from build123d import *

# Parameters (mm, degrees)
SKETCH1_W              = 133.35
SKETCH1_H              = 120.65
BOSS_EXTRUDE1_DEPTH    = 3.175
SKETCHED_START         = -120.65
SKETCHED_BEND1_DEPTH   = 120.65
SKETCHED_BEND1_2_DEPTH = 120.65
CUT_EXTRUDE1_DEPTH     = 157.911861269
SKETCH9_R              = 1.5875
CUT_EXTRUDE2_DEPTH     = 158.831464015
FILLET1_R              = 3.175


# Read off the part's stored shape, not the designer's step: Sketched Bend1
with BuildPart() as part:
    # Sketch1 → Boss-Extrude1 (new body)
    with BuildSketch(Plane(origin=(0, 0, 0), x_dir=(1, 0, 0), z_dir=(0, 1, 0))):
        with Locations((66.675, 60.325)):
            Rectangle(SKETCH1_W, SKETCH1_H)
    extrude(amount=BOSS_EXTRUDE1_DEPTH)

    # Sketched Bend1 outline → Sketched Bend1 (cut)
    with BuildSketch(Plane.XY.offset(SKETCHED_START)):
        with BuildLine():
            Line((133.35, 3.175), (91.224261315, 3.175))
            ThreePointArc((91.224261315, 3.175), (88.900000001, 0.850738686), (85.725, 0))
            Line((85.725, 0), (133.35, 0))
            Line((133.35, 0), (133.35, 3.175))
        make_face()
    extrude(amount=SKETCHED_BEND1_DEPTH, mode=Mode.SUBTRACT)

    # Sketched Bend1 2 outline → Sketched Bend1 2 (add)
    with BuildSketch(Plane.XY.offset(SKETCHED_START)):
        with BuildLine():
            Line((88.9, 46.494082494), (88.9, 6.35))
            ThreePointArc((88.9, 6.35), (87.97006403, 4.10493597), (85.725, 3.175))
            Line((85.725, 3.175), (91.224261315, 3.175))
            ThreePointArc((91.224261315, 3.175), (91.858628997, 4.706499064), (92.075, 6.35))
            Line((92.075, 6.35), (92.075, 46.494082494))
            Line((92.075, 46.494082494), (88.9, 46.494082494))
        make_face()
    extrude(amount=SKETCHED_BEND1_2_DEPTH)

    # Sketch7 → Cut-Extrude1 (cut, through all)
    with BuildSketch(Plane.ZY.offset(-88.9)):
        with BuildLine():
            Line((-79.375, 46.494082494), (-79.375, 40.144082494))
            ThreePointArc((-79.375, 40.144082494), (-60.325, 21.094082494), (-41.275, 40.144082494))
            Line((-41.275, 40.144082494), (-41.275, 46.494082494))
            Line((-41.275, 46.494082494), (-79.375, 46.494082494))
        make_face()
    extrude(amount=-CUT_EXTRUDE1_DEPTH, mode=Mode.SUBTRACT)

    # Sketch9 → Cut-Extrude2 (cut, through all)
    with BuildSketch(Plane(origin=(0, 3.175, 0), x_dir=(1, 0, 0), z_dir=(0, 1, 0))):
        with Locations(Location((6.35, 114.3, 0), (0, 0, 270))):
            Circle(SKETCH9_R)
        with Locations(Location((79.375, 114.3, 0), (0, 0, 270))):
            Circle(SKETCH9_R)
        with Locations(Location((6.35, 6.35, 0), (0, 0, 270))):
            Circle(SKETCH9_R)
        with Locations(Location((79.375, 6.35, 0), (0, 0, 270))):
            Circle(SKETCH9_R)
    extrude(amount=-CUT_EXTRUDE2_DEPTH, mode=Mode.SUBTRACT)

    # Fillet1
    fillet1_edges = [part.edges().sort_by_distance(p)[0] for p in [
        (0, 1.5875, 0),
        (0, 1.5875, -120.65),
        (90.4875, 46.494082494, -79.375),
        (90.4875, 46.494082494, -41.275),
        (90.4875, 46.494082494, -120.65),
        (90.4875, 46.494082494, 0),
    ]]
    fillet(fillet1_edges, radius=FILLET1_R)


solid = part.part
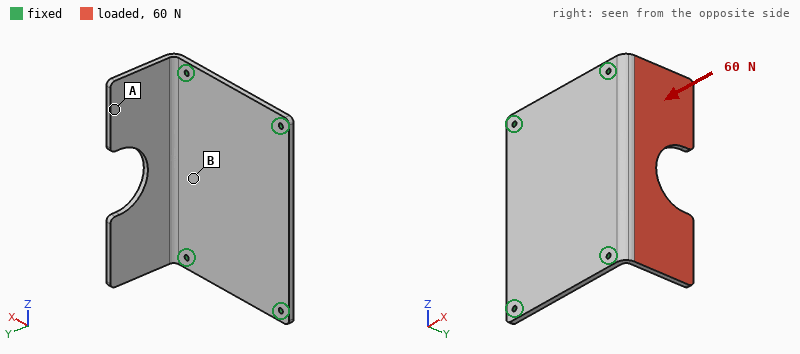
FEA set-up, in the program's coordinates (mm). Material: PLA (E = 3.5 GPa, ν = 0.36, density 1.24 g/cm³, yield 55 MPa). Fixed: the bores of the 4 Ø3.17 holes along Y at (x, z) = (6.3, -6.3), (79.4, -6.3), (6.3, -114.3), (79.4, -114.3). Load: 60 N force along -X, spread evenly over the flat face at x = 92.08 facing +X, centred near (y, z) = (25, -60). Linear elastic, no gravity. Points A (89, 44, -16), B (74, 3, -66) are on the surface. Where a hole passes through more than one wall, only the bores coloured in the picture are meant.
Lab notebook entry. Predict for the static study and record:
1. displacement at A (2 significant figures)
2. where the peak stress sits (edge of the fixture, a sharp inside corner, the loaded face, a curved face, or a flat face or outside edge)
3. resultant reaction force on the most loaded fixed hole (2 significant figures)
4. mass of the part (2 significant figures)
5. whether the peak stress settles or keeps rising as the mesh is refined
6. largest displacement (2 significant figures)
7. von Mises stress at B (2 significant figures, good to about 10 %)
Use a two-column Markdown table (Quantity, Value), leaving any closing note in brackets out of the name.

| Quantity | Value |
|---|---|
| displacement at A | 1.3 mm |
| where the peak stress sits | edge of the fixture |
| resultant reaction force on the most loaded fixed hole | 21 N |
| mass of the part | 60 g |
| whether the peak stress settles or keeps rising as the mesh is refined | keeps rising |
| largest displacement | 1.5 mm |
| von Mises stress at B | 3.4 MPa |
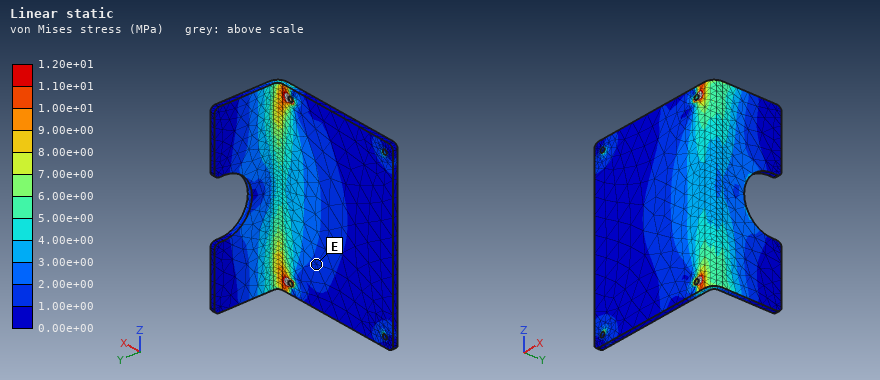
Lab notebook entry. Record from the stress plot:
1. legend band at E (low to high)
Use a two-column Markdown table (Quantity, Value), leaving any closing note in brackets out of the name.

| Quantity | Value |
|---|---|
| legend band at E | 1.00e+00 to 2.00e+00 MPa |
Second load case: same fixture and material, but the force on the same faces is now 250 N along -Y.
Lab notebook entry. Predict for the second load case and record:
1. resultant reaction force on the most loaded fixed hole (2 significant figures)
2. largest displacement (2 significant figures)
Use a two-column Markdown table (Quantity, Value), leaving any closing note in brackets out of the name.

| Quantity | Value |
|---|---|
| resultant reaction force on the most loaded fixed hole | 160 N |
| largest displacement | 1.8 mm |
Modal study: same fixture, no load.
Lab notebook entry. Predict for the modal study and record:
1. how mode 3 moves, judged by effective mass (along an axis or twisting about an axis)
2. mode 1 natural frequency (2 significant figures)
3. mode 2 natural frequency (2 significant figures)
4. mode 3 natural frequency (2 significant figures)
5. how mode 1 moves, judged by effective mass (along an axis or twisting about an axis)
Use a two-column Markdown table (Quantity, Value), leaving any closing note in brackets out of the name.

| Quantity | Value |
|---|---|
| how mode 3 moves, judged by effective mass | along Y |
| mode 1 natural frequency | 310 Hz |
| mode 2 natural frequency | 390 Hz |
| mode 3 natural frequency | 450 Hz |
| how mode 1 moves, judged by effective mass | along X |
